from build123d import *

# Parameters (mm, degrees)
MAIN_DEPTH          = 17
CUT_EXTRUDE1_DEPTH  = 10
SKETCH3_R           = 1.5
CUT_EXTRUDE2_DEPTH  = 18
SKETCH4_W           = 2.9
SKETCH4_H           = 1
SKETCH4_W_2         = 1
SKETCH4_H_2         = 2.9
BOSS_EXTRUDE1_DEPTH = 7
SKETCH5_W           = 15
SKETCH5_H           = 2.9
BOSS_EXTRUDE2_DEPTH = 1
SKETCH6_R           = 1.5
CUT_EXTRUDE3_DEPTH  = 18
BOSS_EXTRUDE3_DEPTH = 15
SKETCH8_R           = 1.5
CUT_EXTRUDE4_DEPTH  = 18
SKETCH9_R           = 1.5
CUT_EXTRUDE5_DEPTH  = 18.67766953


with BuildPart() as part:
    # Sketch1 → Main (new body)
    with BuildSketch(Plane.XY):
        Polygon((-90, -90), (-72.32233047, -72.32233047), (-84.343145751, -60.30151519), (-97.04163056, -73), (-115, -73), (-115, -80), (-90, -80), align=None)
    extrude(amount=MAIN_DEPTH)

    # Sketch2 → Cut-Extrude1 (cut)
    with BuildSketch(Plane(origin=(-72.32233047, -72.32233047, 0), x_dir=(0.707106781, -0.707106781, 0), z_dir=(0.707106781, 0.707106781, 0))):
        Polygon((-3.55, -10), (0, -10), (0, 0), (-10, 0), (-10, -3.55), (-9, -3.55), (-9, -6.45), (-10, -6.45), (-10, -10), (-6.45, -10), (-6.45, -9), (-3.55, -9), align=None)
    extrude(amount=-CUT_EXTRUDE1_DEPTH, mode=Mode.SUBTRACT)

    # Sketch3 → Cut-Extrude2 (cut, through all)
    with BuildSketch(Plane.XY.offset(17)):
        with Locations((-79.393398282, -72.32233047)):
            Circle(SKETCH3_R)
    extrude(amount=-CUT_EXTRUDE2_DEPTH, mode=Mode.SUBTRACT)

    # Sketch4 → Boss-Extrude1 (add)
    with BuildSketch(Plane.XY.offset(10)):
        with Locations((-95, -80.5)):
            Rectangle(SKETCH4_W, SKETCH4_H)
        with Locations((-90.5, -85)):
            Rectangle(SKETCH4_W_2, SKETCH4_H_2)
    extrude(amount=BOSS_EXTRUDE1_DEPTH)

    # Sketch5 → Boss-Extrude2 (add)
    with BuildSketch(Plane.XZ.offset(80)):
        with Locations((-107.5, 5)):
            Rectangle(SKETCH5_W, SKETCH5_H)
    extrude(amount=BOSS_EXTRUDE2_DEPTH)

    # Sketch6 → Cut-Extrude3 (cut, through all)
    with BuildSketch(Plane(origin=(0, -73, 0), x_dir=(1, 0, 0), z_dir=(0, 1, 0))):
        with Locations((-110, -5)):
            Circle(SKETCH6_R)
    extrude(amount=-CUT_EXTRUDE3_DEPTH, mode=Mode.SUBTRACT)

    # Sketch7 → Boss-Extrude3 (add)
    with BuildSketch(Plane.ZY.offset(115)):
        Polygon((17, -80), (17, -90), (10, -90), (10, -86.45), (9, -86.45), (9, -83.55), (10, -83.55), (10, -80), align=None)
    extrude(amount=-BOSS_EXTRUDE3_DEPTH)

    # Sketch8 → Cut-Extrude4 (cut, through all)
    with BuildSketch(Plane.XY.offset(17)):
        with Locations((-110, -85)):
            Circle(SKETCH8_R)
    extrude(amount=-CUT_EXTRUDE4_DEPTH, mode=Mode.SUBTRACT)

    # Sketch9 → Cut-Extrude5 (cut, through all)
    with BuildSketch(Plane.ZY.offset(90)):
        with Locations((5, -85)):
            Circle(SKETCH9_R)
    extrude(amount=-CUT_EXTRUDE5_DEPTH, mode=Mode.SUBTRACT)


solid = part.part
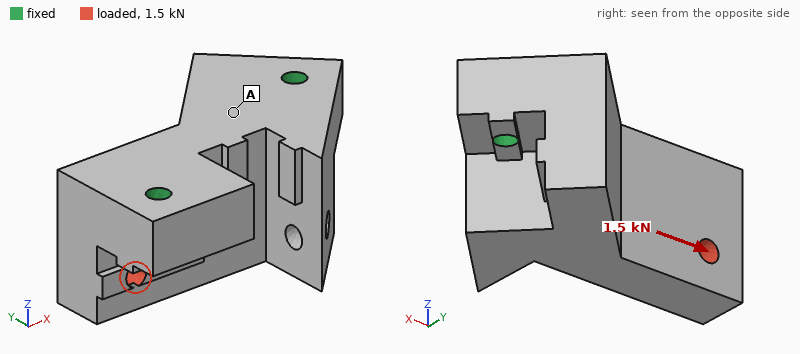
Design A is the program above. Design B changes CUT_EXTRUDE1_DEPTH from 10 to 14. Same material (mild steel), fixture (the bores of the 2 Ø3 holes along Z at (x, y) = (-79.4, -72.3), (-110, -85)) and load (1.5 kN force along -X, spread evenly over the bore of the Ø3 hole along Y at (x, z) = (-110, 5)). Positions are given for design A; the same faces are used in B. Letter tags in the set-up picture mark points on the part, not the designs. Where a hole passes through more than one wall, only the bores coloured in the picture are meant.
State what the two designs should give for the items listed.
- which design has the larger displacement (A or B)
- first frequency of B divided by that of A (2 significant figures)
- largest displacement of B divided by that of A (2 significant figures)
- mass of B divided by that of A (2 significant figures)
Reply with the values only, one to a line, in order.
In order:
B
1.00
1.1
0.95
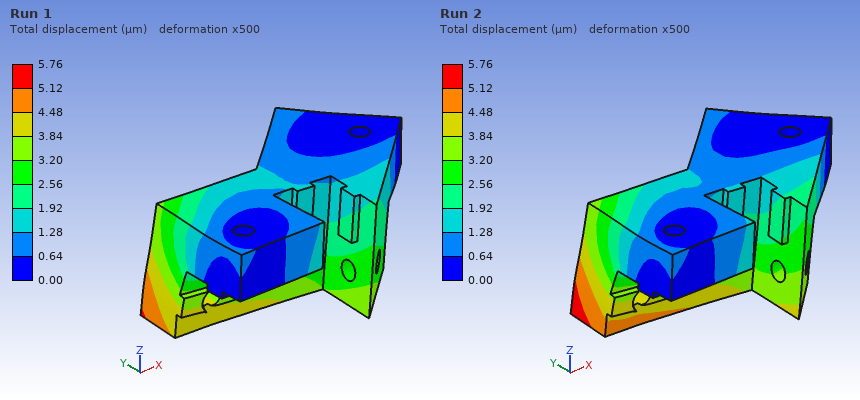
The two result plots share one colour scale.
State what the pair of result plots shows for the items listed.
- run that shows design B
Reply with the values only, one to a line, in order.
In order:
Run 2
